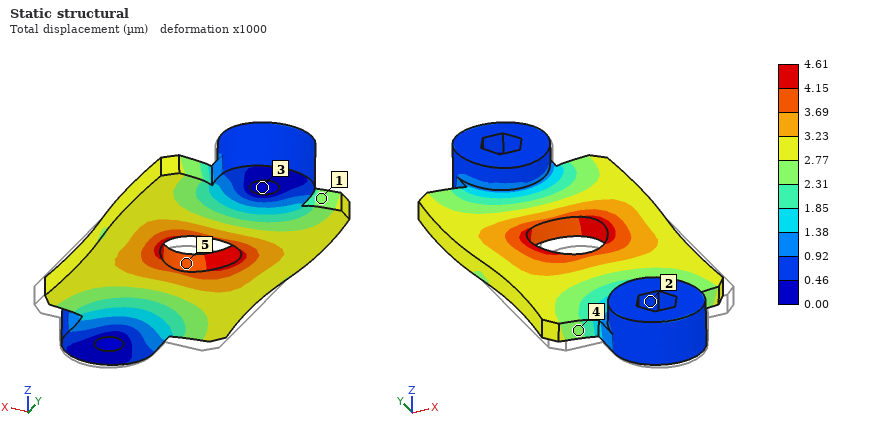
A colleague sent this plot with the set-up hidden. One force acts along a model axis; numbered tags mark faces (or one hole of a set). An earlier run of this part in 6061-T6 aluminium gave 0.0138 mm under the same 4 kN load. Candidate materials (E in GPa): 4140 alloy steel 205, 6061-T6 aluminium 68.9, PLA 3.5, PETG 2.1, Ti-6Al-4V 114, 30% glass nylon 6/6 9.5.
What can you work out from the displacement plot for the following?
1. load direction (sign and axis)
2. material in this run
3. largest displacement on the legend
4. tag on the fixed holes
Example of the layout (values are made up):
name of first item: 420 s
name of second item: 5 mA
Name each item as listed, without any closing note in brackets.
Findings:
load direction: +Y
material in this run: 4140 alloy steel
largest displacement on the legend: 4.61 µm
tag on the fixed holes: 3
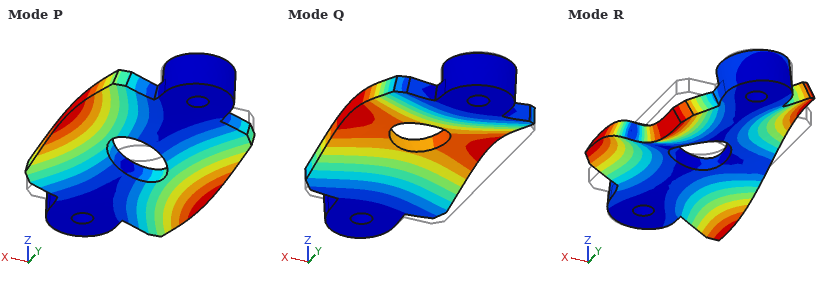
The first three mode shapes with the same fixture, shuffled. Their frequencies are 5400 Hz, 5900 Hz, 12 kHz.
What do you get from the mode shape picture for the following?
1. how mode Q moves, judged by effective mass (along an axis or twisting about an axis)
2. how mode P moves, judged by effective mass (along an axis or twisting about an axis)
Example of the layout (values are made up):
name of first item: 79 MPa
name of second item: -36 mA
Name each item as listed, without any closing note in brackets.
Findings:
how mode Q moves, judged by effective mass: along Z
how mode P moves, judged by effective mass: twisting about Y
